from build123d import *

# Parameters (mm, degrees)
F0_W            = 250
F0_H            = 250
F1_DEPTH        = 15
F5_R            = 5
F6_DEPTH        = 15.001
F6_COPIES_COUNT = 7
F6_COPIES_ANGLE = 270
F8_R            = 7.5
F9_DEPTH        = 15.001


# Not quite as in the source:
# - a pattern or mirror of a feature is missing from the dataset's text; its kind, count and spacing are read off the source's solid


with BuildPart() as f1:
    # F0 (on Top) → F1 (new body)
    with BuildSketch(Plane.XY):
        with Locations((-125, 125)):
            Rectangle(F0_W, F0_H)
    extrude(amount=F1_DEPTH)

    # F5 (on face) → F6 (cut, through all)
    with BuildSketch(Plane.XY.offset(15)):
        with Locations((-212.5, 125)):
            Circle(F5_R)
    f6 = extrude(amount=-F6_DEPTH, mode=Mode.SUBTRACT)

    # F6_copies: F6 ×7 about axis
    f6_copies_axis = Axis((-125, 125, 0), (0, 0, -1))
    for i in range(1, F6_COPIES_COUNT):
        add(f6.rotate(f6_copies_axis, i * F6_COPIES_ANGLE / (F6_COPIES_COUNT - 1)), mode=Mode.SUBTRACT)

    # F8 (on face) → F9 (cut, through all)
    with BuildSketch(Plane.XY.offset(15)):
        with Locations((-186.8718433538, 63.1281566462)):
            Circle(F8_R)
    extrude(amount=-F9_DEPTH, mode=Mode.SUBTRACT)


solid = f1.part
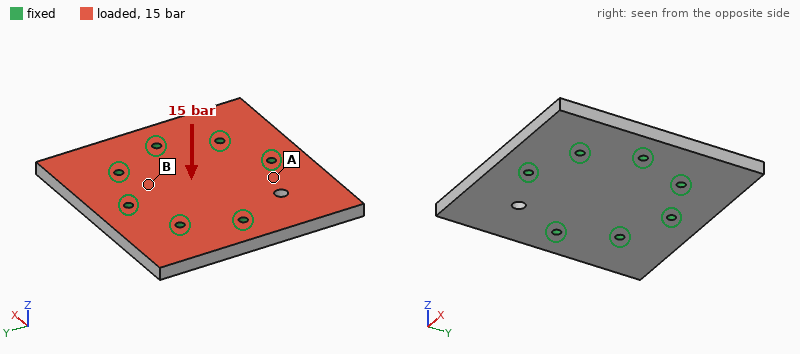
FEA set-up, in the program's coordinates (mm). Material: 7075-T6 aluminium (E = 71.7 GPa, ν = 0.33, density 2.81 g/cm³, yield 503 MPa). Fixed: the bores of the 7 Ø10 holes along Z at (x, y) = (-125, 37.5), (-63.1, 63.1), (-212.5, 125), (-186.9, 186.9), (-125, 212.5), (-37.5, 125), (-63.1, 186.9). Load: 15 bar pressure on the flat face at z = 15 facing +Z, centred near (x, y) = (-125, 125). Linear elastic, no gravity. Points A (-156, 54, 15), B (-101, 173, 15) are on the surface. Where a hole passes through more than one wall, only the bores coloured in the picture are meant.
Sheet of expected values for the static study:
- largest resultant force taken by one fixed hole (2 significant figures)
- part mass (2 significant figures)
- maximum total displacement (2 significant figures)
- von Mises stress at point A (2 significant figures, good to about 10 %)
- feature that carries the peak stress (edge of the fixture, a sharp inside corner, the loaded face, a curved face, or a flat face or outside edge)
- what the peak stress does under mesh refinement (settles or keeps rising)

18 kN
2.6 kg
0.89 mm
64 MPa
edge of the fixture
keeps rising
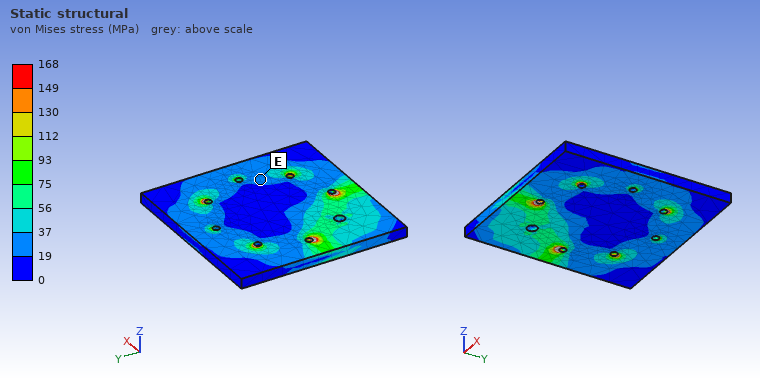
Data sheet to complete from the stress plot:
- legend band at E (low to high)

19 to 37 MPa
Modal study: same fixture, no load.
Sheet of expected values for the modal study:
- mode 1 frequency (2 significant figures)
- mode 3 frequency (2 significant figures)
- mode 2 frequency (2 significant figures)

1400 Hz
2300 Hz
2300 Hz
